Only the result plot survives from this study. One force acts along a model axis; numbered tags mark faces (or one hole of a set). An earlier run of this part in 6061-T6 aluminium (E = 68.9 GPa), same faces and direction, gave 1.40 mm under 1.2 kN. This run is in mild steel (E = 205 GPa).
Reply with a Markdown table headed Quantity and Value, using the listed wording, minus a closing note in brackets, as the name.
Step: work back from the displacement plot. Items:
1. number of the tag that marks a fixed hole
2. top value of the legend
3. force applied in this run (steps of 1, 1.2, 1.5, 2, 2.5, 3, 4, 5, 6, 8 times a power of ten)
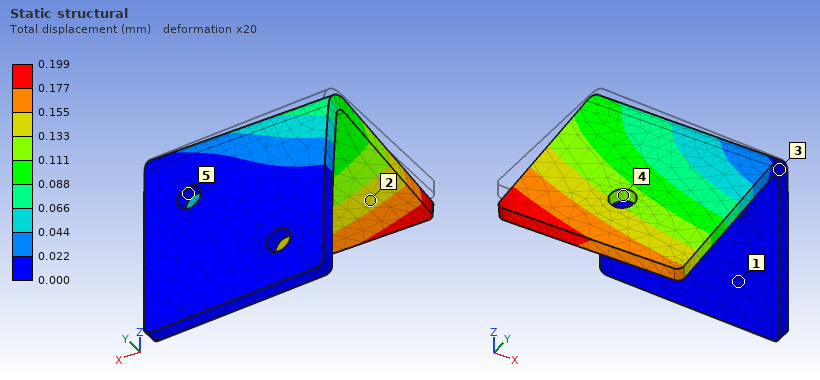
| Quantity | Value |
|---|---|
| number of the tag that marks a fixed hole | 5 |
| top value of the legend | 0.199 mm |
| force applied in this run | 500 N |
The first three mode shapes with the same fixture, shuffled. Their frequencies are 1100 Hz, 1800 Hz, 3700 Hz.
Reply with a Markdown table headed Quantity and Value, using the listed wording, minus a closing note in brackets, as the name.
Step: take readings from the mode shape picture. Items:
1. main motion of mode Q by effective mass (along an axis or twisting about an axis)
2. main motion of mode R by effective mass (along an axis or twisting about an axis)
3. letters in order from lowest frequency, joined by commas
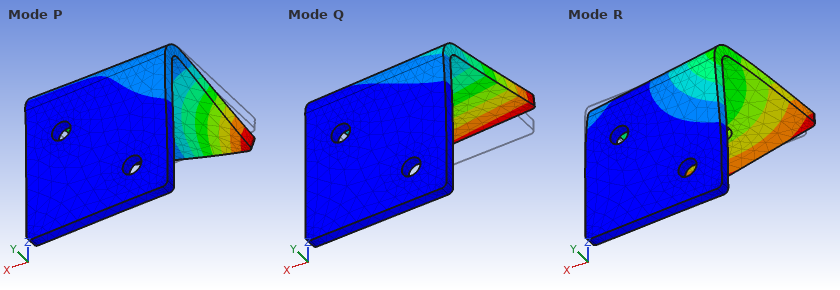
| Quantity | Value |
|---|---|
| main motion of mode Q by effective mass | along Z |
| main motion of mode R by effective mass | along X |
| letters in order from lowest frequency, joined by commas | Q, R, P |
